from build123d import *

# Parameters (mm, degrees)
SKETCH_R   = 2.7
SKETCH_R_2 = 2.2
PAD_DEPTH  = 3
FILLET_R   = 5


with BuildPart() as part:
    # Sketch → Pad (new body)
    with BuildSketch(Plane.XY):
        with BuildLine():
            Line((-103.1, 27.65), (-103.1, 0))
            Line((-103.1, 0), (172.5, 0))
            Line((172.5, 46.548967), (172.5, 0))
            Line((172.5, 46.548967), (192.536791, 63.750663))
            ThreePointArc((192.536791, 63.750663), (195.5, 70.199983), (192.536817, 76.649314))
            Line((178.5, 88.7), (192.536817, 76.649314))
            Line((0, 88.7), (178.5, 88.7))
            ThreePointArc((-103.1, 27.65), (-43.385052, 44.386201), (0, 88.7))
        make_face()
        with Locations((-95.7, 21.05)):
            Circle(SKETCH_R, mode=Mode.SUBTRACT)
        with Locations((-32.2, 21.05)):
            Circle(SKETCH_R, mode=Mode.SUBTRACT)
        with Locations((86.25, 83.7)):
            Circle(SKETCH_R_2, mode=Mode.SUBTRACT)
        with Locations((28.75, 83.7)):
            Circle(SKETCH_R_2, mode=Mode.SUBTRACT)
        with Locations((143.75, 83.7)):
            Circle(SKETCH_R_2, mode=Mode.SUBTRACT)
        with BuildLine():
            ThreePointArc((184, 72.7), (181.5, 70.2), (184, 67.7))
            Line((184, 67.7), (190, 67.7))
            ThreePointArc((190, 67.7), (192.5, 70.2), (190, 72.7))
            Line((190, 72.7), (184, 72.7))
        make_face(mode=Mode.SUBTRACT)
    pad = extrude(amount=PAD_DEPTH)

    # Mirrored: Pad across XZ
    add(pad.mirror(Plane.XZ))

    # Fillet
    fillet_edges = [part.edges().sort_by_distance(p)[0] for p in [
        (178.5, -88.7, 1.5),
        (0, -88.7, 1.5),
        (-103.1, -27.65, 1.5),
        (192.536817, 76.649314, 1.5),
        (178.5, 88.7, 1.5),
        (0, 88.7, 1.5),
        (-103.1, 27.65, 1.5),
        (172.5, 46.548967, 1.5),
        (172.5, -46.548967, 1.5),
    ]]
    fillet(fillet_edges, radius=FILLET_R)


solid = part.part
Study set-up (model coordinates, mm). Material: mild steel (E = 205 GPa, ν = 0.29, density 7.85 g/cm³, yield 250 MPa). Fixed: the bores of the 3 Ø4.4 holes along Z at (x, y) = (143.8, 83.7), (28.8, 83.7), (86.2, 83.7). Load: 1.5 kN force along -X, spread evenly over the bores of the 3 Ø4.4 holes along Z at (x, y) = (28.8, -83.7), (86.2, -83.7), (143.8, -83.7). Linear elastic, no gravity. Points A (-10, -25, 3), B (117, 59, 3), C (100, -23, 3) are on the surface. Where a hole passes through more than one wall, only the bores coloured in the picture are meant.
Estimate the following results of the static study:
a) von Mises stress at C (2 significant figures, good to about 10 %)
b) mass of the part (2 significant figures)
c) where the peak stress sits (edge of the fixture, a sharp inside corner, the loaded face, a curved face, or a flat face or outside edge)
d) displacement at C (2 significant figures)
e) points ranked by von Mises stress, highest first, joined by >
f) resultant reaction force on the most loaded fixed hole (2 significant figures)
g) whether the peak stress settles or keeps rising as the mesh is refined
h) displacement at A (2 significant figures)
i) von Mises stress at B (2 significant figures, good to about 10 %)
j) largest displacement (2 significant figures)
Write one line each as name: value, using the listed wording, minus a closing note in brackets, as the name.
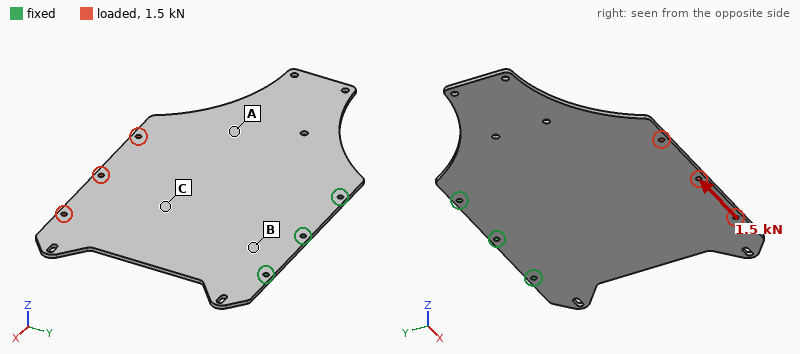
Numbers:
von Mises stress at C: 7.2 MPa
mass of the part: 960 g
where the peak stress sits: edge of the fixture
displacement at C: 16 µm
points ranked by von Mises stress, highest first, joined by >: B > C > A
resultant reaction force on the most loaded fixed hole: 2.2 kN
whether the peak stress settles or keeps rising as the mesh is refined: keeps rising
displacement at A: 20 µm
von Mises stress at B: 12 MPa
largest displacement: 30 µm
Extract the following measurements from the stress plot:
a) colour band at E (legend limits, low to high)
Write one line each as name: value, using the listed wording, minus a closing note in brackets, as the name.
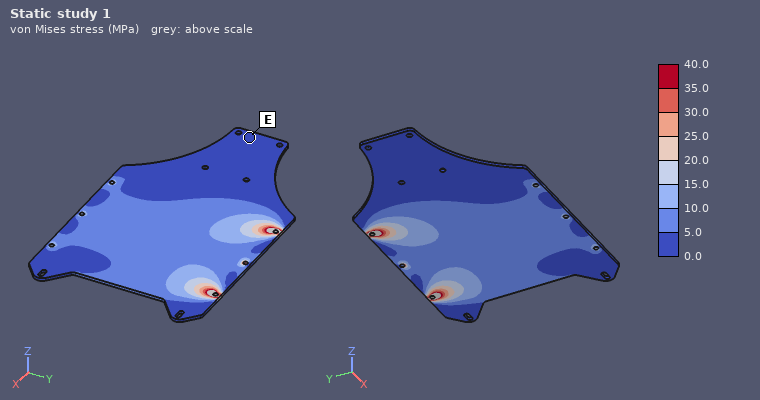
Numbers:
colour band at E: 0.0 to 5.0 MPa
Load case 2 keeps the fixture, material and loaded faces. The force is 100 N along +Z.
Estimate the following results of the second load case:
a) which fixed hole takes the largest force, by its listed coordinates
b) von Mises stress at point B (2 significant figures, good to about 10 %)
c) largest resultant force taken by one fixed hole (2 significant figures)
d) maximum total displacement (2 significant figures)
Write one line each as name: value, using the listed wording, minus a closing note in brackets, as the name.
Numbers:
which fixed hole takes the largest force, by its listed coordinates: (86.2, 83.7)
von Mises stress at point B: 46 MPa
largest resultant force taken by one fixed hole: 58 N
maximum total displacement: 2.1 mm
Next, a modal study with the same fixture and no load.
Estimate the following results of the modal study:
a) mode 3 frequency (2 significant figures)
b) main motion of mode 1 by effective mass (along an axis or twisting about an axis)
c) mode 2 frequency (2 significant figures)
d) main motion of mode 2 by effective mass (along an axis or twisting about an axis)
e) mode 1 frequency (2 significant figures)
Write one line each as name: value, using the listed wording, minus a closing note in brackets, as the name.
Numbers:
mode 3 frequency: 250 Hz
main motion of mode 1 by effective mass: along Z
mode 2 frequency: 120 Hz
main motion of mode 2 by effective mass: twisting about Y
mode 1 frequency: 71 Hz
